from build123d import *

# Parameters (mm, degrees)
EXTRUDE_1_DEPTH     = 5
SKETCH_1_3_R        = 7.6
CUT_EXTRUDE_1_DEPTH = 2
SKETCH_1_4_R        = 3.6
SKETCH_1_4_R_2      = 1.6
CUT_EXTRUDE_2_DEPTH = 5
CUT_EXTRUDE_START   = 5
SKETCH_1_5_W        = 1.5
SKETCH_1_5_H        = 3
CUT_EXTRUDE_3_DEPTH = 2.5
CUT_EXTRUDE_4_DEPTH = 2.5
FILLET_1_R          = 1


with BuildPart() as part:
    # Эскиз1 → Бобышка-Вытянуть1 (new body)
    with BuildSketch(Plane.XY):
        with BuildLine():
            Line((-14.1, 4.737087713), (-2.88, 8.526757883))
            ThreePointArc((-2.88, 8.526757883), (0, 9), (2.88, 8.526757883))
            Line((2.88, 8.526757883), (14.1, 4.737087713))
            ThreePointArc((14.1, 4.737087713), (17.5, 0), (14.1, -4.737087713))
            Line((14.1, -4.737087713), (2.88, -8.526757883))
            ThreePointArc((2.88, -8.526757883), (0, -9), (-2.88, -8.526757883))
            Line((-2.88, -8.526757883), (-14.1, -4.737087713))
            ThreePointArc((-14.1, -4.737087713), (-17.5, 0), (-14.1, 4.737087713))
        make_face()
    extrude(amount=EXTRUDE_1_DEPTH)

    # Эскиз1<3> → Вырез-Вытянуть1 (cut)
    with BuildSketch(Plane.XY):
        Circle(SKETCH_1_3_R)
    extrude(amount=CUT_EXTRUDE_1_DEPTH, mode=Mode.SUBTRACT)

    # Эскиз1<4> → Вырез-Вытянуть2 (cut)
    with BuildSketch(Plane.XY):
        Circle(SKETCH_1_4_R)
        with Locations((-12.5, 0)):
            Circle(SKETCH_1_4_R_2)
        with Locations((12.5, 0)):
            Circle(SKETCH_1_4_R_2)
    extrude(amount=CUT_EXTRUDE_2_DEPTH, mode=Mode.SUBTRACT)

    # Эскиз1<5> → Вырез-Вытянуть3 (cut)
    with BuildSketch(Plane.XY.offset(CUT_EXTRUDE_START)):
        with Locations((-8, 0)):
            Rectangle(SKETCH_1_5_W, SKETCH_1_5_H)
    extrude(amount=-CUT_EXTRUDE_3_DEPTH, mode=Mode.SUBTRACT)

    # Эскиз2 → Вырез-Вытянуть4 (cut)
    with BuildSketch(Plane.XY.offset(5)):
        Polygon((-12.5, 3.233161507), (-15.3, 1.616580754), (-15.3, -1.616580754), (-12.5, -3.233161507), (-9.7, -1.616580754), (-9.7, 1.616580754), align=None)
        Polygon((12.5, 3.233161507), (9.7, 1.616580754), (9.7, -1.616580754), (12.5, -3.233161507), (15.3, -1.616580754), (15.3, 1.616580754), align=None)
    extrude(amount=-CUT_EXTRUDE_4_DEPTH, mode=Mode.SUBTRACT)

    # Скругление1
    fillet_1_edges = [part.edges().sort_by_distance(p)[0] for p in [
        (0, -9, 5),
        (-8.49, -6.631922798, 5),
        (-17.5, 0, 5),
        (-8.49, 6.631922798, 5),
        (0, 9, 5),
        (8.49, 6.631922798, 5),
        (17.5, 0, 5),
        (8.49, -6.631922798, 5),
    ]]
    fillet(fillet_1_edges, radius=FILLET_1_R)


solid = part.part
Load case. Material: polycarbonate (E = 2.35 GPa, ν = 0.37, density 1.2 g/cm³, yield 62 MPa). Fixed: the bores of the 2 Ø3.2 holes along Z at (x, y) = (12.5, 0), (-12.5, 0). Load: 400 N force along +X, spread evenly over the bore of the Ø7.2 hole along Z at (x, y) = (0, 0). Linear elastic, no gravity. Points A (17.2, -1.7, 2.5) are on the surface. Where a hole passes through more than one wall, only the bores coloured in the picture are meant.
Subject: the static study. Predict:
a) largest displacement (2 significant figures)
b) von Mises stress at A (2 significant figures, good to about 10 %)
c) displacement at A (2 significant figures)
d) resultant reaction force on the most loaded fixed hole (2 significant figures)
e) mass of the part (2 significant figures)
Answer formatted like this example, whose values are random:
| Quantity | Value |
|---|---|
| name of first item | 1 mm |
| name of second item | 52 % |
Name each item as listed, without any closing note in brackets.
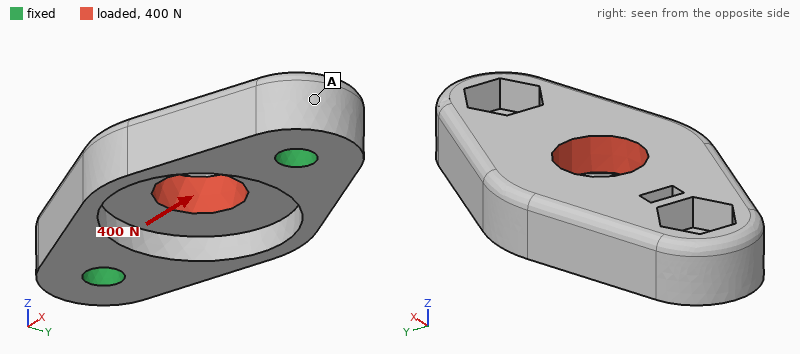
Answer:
| Quantity | Value |
|---|---|
| largest displacement | 48 µm |
| von Mises stress at A | 2.8 MPa |
| displacement at A | 16 µm |
| resultant reaction force on the most loaded fixed hole | 200 N |
| mass of the part | 1.9 g |
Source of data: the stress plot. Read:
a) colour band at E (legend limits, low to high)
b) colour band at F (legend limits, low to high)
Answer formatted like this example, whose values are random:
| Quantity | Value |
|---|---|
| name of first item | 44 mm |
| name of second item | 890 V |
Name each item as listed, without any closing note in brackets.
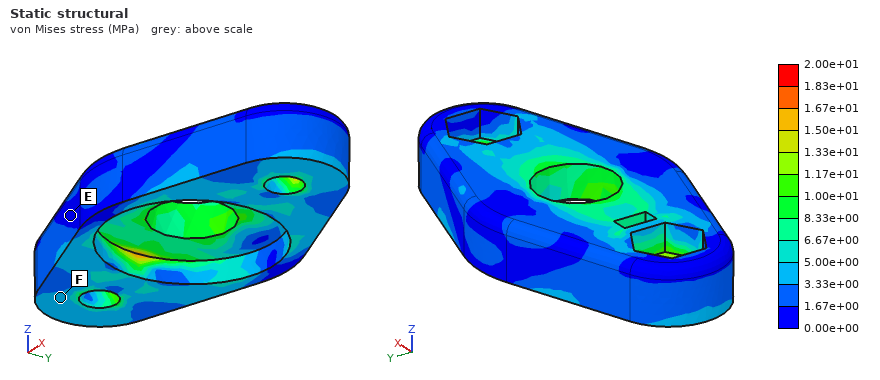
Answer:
| Quantity | Value |
|---|---|
| colour band at E | 0.00e+00 to 1.67e+00 MPa |
| colour band at F | 3.33e+00 to 5.00e+00 MPa |
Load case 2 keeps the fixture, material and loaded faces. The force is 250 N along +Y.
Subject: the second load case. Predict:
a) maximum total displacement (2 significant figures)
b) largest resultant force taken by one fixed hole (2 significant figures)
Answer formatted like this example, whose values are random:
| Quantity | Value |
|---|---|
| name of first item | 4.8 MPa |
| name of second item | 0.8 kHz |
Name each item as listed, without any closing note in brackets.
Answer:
| Quantity | Value |
|---|---|
| maximum total displacement | 0.14 mm |
| largest resultant force taken by one fixed hole | 130 N |
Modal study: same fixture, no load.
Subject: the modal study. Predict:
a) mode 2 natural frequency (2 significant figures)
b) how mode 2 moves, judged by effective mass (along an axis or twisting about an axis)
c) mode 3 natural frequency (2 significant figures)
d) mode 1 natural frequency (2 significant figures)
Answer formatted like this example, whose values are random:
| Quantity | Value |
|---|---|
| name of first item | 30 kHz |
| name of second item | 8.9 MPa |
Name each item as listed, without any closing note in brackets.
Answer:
| Quantity | Value |
|---|---|
| mode 2 natural frequency | 6800 Hz |
| how mode 2 moves, judged by effective mass | along Z |
| mode 3 natural frequency | 13 kHz |
| mode 1 natural frequency | 5300 Hz |
